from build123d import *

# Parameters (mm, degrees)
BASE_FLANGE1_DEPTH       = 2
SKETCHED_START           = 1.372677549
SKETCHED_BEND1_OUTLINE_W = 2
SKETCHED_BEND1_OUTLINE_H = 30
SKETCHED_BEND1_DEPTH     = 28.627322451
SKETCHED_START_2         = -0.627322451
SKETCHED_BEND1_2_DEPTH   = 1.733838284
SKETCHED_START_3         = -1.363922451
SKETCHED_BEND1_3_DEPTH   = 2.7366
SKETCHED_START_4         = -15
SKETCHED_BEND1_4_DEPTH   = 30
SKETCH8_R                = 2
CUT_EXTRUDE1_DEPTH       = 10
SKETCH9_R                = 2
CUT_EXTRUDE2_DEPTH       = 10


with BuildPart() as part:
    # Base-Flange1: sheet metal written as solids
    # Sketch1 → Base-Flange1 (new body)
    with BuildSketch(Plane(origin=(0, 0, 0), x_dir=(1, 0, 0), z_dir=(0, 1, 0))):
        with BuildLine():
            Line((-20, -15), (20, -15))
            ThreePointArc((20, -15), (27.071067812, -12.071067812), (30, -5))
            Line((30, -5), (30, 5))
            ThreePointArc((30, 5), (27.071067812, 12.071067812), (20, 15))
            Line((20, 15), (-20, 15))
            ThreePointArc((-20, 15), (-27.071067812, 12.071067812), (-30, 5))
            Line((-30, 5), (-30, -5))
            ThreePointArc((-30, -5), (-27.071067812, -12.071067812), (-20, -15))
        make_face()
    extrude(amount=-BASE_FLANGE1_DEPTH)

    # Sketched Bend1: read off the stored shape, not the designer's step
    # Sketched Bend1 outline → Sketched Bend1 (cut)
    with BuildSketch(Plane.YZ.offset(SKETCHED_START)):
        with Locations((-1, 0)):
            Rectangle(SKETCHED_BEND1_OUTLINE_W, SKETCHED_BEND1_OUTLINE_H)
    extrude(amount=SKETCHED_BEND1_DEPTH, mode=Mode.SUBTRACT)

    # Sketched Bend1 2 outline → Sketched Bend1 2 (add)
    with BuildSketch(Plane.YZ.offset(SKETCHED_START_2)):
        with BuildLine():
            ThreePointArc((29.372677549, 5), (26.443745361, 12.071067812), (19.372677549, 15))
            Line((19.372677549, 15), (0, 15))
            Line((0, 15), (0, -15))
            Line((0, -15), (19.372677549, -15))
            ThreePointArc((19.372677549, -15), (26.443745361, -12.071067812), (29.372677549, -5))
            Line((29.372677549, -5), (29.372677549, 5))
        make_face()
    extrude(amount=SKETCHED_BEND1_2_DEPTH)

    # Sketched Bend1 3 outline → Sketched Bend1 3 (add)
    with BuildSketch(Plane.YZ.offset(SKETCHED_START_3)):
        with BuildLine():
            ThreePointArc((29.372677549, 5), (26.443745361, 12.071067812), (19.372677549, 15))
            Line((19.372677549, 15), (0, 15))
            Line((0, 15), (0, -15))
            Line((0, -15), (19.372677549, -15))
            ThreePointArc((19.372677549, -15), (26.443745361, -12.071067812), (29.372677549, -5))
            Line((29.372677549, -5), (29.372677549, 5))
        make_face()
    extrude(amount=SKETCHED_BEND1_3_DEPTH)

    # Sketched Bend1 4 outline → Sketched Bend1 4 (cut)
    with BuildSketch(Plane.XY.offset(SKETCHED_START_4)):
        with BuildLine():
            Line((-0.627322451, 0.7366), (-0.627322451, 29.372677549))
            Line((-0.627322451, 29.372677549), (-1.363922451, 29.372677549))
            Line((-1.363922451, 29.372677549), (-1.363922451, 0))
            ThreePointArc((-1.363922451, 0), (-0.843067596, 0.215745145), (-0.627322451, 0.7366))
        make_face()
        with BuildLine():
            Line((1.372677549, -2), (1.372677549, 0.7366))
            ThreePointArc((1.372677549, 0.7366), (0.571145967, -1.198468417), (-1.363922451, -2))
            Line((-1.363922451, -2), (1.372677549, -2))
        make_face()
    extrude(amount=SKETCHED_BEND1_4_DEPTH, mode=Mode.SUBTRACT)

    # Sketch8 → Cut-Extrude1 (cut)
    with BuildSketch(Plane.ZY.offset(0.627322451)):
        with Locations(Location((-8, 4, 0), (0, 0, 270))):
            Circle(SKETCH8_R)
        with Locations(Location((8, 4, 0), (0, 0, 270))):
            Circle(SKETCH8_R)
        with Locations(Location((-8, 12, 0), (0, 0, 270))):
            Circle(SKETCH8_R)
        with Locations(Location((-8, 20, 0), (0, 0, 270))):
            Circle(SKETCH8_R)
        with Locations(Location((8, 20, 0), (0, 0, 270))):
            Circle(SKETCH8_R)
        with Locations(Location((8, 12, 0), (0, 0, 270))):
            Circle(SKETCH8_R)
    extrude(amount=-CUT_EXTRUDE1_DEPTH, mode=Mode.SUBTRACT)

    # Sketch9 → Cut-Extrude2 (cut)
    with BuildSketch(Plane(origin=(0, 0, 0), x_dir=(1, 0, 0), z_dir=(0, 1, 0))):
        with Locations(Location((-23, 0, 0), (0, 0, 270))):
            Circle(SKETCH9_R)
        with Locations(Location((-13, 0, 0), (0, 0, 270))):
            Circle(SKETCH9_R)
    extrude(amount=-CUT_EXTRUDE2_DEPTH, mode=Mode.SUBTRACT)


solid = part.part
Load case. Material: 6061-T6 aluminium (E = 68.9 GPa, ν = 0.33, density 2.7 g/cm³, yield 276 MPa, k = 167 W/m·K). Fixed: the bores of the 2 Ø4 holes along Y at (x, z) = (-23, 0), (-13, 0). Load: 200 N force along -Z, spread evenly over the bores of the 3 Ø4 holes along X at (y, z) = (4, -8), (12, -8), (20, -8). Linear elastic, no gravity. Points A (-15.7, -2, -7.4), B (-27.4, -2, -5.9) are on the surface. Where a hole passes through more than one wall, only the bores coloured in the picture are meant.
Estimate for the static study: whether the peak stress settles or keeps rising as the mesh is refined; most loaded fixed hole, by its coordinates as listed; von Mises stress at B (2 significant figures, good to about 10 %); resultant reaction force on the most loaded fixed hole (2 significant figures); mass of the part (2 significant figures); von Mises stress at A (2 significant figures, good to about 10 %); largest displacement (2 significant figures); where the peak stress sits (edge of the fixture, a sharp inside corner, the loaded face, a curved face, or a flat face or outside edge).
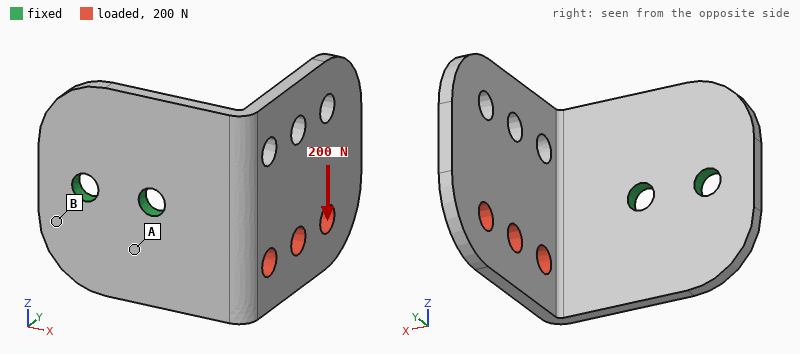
keeps rising
(-13, 0)
22 MPa
370 N
8.7 g
69 MPa
0.44 mm
edge of the fixture
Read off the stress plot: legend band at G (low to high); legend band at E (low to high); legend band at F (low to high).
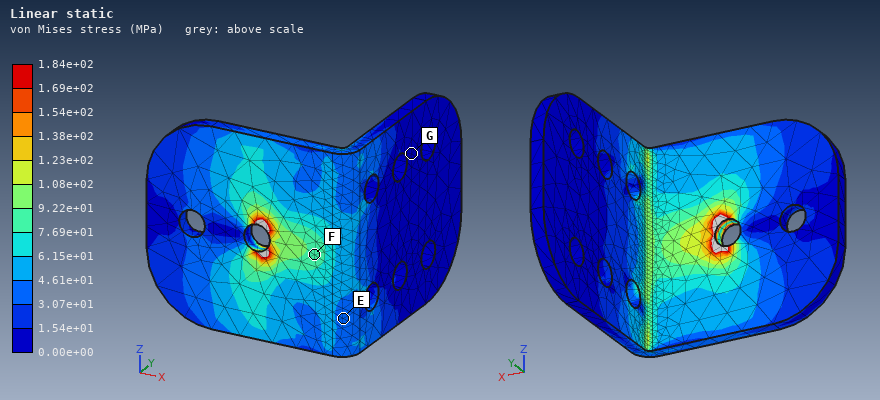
0.00e+00 to 1.54e+01 MPa
3.07e+01 to 4.61e+01 MPa
7.69e+01 to 9.22e+01 MPa
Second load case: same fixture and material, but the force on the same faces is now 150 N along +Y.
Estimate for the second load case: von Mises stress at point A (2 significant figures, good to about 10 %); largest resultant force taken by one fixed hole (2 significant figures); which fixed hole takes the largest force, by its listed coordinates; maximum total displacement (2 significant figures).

55 MPa
210 N
(-13, 0)
0.39 mm
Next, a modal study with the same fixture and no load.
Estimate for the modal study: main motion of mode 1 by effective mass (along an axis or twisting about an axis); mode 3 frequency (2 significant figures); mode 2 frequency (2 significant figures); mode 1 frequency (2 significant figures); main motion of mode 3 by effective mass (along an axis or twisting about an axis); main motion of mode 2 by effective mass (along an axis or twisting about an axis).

along X
3900 Hz
1700 Hz
1100 Hz
along Y
along Z
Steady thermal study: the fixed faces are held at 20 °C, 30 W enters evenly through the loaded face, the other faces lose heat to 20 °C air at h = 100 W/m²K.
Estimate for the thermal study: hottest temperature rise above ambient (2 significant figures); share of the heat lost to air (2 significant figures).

74 K
37 %
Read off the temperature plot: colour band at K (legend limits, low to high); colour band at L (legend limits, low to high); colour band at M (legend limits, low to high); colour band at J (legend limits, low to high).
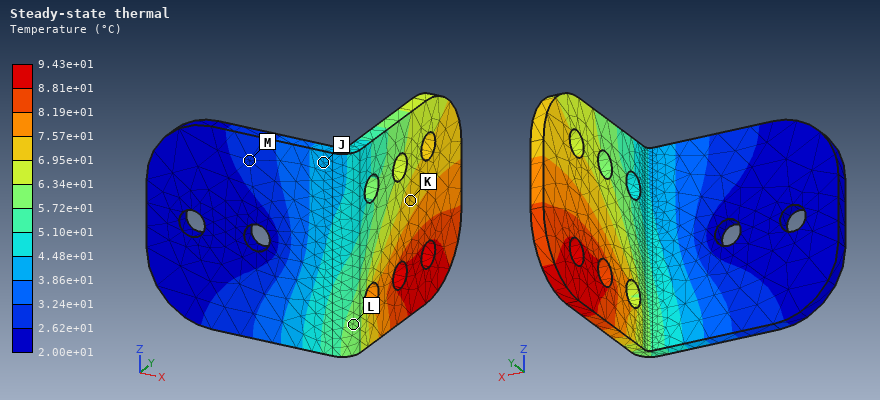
6.95e+01 to 7.57e+01 °C
5.72e+01 to 6.34e+01 °C
2.62e+01 to 3.24e+01 °C
3.86e+01 to 4.48e+01 °C
